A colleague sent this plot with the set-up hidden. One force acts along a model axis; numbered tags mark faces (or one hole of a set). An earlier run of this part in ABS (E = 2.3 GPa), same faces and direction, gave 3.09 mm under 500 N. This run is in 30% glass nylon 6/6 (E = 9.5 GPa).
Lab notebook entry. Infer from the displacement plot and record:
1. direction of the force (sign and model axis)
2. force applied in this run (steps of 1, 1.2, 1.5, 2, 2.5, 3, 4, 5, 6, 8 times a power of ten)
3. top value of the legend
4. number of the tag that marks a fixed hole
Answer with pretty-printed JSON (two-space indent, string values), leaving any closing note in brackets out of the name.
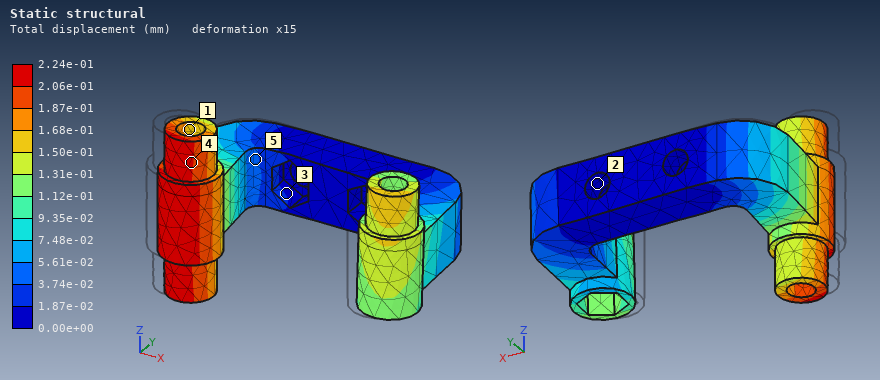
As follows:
{
  "direction of the force": "+X",
  "force applied in this run": "150 N",
  "top value of the legend": "2.24e-01 mm",
  "number of the tag that marks a fixed hole": "2"
}
